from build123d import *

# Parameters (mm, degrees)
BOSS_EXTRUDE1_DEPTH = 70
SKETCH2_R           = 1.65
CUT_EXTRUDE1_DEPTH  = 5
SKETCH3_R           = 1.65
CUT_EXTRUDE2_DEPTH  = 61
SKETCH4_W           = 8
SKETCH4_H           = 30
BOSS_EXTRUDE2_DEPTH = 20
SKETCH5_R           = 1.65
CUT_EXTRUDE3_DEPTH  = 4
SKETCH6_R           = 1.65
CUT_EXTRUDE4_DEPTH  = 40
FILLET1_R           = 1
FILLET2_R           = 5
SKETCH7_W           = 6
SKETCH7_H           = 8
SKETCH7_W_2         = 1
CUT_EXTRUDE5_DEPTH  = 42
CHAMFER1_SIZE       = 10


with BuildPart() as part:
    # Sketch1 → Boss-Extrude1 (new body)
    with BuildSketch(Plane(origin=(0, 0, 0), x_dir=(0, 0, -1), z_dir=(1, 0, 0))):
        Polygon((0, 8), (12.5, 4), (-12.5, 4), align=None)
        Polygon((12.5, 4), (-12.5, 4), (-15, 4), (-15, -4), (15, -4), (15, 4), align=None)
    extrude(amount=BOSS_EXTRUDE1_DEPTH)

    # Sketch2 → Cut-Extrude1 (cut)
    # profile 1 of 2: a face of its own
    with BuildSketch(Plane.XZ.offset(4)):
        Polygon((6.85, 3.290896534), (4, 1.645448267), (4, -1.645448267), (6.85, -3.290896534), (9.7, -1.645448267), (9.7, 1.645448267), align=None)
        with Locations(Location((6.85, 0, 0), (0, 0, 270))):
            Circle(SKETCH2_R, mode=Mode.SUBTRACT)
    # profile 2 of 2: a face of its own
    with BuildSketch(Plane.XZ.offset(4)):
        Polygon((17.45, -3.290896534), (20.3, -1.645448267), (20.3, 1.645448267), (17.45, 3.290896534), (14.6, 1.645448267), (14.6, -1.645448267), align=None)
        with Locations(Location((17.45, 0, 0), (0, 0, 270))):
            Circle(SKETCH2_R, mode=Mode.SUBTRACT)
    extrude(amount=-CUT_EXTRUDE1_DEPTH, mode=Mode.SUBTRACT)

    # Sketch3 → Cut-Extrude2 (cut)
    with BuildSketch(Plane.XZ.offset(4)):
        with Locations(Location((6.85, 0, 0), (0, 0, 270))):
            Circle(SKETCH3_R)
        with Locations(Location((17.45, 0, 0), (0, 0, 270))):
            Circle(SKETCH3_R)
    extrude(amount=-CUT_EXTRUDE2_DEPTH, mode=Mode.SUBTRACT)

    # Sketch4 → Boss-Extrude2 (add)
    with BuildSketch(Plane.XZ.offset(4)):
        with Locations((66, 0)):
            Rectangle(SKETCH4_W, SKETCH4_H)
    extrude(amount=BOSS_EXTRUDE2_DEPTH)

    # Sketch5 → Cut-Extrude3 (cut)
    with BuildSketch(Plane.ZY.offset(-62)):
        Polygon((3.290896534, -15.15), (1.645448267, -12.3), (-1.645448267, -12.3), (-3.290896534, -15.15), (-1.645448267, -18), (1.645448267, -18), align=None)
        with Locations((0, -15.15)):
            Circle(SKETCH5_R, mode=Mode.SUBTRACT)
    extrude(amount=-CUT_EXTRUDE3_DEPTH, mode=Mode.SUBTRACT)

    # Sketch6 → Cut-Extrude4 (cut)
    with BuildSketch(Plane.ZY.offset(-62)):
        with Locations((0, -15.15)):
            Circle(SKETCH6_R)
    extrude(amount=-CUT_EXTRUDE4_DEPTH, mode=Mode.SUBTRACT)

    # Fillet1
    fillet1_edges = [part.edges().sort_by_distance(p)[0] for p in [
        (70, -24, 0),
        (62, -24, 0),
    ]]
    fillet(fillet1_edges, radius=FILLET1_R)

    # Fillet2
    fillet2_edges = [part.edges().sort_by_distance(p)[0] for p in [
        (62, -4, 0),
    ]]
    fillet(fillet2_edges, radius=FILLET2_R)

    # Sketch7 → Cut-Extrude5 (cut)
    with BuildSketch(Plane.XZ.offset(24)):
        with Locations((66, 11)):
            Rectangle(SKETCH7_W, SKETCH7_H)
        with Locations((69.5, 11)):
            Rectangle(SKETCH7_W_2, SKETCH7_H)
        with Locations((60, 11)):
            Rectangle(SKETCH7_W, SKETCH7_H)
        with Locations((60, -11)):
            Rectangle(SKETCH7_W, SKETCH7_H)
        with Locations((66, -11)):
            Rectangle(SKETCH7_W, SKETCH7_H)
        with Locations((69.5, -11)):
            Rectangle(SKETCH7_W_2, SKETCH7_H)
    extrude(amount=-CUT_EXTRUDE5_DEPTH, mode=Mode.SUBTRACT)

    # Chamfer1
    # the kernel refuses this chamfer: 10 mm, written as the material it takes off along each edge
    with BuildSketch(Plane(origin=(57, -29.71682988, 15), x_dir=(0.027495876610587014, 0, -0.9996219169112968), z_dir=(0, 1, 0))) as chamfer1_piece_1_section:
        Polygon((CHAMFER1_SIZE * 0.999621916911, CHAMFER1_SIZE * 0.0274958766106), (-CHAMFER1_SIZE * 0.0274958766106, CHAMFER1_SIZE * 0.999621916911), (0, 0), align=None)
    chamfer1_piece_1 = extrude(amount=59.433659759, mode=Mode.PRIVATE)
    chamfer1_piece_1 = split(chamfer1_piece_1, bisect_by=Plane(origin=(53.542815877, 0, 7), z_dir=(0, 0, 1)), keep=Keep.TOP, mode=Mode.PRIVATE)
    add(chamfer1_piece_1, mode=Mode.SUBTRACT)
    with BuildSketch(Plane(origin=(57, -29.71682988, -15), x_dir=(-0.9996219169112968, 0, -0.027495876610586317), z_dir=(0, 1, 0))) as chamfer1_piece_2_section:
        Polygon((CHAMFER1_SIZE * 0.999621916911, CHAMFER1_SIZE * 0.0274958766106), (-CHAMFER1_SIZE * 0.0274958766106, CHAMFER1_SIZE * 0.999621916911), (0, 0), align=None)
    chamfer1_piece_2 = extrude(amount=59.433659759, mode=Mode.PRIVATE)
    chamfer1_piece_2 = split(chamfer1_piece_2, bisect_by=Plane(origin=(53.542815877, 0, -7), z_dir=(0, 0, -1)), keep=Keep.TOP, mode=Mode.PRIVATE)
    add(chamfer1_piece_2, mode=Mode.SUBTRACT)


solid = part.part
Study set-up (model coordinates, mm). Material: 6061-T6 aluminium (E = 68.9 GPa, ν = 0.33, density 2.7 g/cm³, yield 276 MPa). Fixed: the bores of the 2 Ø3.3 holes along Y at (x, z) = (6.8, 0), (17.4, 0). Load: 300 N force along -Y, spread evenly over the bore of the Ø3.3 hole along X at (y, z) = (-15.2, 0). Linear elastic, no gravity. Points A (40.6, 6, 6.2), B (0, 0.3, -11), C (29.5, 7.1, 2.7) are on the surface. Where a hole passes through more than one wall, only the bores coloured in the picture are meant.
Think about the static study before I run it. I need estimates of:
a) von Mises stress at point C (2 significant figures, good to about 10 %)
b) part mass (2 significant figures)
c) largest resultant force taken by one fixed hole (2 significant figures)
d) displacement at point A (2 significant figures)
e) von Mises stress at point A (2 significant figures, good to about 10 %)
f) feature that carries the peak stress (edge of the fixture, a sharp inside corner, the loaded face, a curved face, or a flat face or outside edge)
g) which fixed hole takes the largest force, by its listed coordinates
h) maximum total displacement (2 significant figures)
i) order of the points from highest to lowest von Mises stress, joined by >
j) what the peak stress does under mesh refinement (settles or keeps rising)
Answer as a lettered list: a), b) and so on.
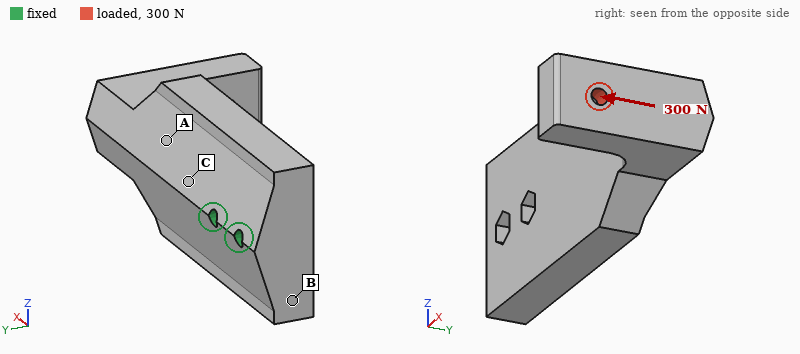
a) 28 MPa
b) 53 g
c) 1.2 kN
d) 0.035 mm
e) 17 MPa
f) edge of the fixture
g) (17.4, 0)
h) 0.14 mm
i) C > A > B
j) keeps rising
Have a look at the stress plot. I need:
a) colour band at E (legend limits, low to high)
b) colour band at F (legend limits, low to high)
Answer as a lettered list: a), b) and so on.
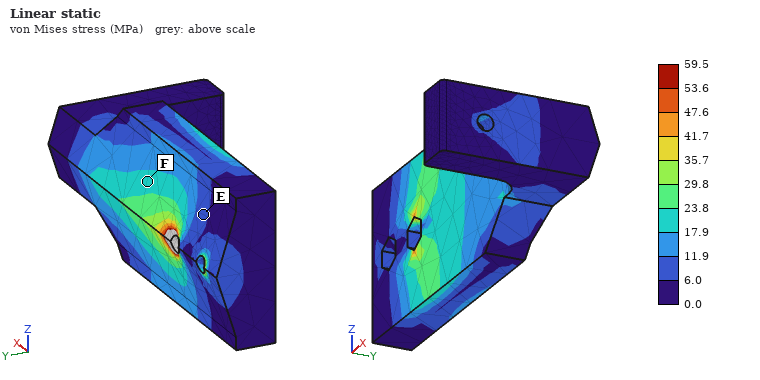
a) 6.0 to 11.9 MPa
b) 17.9 to 23.8 MPa
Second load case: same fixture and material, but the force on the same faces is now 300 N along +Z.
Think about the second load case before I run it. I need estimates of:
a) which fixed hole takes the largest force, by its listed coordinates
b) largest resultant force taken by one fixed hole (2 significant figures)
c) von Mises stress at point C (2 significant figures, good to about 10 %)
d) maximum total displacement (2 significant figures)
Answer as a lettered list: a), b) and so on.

a) (17.4, 0)
b) 1.4 kN
c) 8.7 MPa
d) 92 µm
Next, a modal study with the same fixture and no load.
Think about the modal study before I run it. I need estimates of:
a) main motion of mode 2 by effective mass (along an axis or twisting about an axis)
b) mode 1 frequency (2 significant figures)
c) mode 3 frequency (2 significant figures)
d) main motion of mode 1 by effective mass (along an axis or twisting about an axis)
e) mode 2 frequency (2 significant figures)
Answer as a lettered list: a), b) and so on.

a) along Z
b) 2300 Hz
c) 6900 Hz
d) along Y
e) 3500 Hz
